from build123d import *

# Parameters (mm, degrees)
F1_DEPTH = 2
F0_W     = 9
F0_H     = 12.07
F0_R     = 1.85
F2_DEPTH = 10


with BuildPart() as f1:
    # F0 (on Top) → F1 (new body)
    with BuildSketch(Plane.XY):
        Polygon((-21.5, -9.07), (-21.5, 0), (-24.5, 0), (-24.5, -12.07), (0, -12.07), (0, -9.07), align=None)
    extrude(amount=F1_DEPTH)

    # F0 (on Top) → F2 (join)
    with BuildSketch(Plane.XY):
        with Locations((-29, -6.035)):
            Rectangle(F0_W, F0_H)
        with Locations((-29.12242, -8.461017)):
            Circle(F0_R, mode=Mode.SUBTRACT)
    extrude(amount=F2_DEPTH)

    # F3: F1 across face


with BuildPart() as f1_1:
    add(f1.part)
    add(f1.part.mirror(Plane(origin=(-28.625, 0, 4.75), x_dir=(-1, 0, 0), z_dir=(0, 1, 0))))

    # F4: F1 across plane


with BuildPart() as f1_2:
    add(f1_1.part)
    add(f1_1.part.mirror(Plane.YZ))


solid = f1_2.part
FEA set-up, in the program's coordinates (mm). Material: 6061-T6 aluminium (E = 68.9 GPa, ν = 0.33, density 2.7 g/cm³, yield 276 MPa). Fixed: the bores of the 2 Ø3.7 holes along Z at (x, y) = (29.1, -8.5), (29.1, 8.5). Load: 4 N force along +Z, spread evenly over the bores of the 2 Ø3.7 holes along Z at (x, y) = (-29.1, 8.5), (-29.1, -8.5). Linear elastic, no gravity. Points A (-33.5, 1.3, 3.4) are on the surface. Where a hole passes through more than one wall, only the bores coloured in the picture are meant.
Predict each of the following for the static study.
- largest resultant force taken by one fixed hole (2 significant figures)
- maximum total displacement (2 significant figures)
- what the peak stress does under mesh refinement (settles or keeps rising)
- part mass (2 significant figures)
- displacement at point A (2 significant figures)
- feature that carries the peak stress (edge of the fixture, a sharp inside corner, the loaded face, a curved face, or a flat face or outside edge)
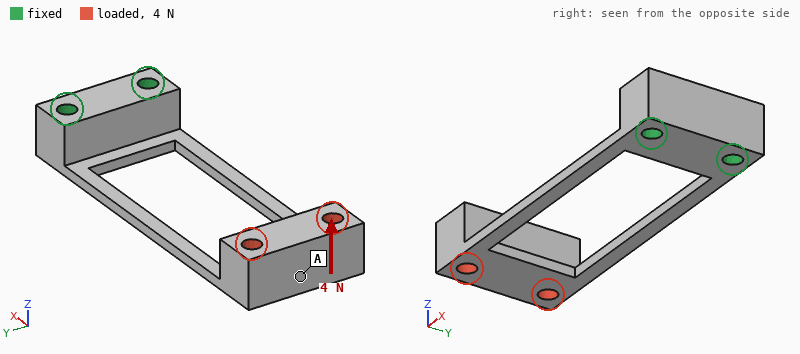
2.1 N
0.84 mm
keeps rising
13 g
0.82 mm
a sharp inside corner
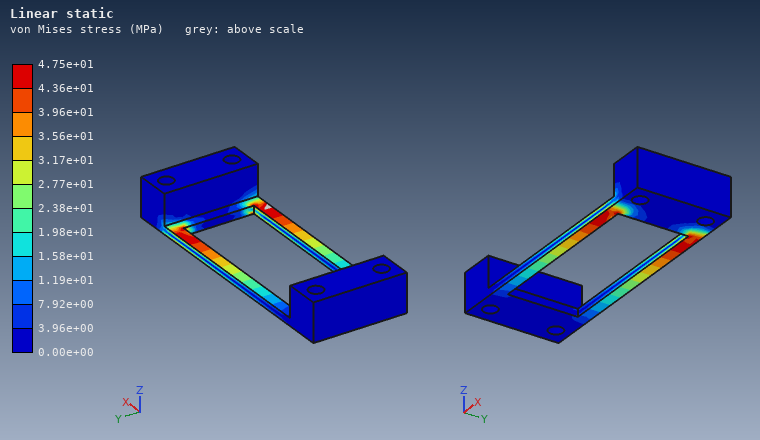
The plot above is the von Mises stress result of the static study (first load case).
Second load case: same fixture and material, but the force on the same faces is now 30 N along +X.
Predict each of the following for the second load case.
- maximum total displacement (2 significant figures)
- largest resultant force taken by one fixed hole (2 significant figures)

0.73 mm
15 N
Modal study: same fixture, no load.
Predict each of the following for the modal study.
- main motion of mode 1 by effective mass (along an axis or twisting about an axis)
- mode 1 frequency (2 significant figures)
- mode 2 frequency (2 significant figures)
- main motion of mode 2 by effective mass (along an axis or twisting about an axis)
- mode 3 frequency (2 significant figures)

along Z
150 Hz
500 Hz
along Y
830 Hz
